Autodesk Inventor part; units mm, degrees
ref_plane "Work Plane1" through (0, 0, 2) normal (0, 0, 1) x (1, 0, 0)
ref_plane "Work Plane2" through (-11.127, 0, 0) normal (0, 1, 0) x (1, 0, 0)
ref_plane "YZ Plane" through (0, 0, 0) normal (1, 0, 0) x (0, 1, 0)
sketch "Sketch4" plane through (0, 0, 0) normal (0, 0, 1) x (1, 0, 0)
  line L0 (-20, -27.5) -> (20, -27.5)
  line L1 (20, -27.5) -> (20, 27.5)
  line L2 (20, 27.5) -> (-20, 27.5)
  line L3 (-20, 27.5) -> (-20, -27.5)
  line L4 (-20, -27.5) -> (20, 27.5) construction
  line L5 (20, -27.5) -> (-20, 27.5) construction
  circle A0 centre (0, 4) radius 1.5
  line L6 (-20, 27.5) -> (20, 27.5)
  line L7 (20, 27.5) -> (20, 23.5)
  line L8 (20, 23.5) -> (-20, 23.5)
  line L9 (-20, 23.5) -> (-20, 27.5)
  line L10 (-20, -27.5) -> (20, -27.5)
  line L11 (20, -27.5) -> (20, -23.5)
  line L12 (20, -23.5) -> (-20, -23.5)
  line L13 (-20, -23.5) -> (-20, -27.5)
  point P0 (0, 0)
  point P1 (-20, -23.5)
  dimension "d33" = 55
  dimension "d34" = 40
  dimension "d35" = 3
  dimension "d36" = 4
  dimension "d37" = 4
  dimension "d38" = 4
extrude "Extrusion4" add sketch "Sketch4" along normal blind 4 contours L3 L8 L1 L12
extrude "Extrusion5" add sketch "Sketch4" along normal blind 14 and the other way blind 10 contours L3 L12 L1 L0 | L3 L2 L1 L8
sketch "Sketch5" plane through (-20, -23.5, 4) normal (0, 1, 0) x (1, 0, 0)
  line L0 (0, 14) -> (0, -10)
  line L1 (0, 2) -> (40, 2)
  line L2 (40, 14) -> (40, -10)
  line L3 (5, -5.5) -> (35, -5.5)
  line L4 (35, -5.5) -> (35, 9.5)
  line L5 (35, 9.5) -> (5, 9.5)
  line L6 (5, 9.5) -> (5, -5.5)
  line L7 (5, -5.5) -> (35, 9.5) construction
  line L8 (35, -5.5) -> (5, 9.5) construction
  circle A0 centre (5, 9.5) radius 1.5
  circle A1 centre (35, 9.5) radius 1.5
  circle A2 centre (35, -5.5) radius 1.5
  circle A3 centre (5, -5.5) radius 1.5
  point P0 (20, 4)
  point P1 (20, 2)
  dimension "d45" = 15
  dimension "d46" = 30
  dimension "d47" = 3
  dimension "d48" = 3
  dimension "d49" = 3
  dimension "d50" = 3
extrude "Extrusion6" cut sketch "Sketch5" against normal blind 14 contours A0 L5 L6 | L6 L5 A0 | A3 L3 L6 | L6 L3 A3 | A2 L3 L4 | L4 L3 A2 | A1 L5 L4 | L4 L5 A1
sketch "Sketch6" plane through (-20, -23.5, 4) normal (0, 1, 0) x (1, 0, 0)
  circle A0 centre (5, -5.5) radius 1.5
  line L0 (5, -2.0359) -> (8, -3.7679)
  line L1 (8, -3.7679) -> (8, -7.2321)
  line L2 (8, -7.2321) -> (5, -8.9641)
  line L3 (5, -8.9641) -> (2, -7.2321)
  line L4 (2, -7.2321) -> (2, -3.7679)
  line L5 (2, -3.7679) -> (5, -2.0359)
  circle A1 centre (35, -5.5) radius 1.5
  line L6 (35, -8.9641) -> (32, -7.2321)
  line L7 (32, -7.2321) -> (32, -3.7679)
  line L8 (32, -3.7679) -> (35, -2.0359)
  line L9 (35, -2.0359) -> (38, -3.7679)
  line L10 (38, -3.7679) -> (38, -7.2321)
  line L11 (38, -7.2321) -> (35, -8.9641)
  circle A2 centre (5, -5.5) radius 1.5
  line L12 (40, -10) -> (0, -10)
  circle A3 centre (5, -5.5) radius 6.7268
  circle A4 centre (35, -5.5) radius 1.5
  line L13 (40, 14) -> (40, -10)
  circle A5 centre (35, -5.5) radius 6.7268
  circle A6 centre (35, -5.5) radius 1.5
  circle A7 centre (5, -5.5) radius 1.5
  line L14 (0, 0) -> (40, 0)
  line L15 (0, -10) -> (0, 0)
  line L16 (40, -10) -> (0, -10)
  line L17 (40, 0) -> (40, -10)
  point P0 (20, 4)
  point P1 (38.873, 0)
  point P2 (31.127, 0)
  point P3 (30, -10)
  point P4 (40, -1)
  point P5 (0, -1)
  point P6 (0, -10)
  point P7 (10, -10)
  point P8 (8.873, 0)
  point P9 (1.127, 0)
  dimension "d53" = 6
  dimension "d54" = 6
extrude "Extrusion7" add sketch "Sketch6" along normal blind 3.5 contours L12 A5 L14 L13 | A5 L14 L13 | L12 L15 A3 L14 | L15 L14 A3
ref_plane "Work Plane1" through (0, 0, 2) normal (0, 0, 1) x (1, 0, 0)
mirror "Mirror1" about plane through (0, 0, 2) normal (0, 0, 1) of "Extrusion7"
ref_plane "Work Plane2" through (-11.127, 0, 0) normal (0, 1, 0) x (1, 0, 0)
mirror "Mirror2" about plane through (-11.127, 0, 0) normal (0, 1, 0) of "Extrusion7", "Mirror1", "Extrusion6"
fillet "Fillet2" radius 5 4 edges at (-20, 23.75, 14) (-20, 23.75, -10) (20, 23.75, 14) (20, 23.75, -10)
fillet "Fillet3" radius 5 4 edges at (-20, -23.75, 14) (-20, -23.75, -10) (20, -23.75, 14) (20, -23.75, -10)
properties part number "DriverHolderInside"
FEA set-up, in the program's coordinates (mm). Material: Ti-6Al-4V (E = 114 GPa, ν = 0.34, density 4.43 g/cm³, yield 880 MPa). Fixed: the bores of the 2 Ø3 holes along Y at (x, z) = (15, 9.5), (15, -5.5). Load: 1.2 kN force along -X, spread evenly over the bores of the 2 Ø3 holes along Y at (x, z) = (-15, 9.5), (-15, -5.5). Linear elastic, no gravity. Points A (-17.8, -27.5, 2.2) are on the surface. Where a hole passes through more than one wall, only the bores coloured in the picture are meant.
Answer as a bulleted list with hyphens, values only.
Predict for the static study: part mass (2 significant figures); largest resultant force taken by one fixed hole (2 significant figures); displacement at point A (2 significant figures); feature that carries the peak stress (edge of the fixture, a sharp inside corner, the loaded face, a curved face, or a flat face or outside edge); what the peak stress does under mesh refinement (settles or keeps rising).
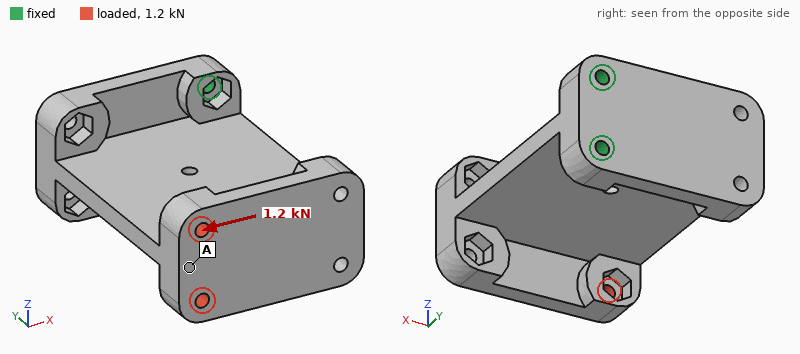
- 75 g
- 690 N
- 0.71 mm
- edge of the fixture
- keeps rising
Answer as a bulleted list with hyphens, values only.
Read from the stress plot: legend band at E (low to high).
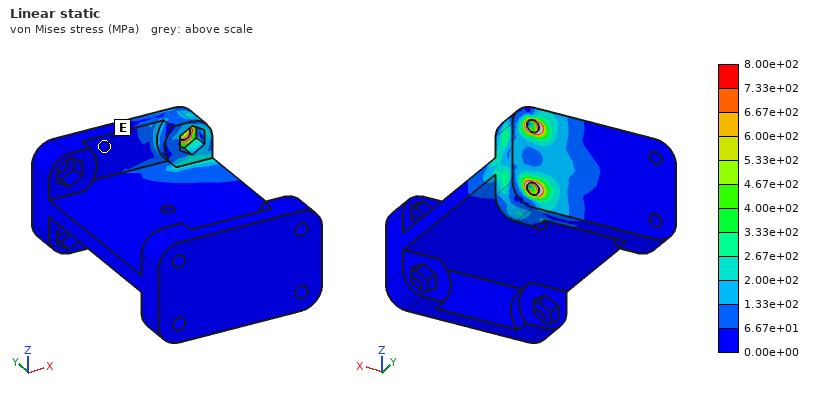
- 0.00e+00 to 6.67e+01 MPa
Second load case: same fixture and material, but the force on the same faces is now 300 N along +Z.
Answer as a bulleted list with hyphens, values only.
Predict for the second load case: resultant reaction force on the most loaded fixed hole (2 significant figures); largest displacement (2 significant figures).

- 1.2 kN
- 0.74 mm
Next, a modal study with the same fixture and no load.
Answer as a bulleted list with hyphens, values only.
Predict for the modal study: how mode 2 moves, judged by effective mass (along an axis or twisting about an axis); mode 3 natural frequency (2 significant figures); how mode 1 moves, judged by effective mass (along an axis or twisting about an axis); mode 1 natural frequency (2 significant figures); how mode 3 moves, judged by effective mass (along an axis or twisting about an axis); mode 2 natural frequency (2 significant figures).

- along X
- 2200 Hz
- along Z
- 700 Hz
- twisting about Y
- 1100 Hz
